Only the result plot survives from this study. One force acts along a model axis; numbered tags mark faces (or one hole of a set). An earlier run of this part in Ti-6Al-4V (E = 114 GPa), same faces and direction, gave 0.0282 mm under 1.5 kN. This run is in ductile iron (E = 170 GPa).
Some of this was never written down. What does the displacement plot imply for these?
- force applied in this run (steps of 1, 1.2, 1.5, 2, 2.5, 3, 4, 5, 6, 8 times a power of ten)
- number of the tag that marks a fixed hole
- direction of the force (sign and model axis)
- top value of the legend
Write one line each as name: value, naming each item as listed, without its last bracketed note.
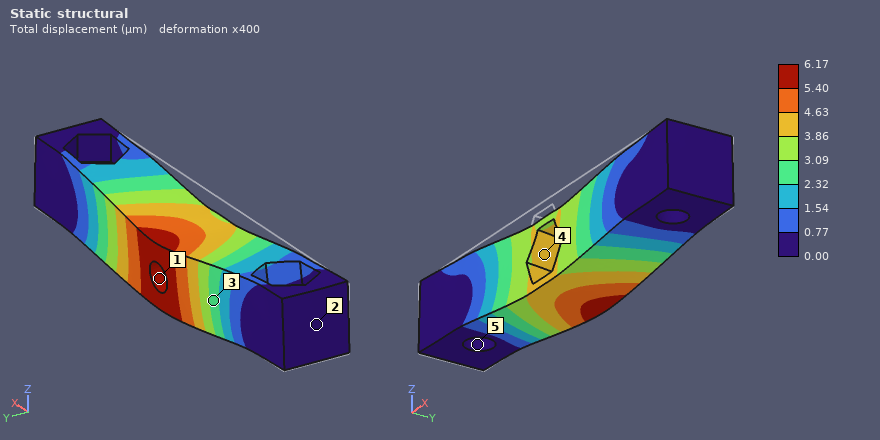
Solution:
force applied in this run: 500 N
number of the tag that marks a fixed hole: 5
direction of the force: -Z
top value of the legend: 6.17 µm
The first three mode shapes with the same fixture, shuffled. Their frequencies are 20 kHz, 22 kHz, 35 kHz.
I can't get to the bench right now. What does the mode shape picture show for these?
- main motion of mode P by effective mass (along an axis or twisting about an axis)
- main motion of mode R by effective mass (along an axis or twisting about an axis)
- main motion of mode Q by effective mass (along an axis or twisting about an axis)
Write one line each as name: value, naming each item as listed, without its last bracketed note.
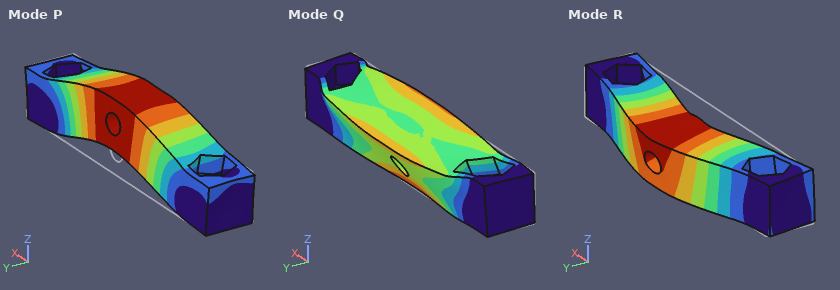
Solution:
main motion of mode P by effective mass: along Z
main motion of mode R by effective mass: along Y
main motion of mode Q by effective mass: twisting about X
